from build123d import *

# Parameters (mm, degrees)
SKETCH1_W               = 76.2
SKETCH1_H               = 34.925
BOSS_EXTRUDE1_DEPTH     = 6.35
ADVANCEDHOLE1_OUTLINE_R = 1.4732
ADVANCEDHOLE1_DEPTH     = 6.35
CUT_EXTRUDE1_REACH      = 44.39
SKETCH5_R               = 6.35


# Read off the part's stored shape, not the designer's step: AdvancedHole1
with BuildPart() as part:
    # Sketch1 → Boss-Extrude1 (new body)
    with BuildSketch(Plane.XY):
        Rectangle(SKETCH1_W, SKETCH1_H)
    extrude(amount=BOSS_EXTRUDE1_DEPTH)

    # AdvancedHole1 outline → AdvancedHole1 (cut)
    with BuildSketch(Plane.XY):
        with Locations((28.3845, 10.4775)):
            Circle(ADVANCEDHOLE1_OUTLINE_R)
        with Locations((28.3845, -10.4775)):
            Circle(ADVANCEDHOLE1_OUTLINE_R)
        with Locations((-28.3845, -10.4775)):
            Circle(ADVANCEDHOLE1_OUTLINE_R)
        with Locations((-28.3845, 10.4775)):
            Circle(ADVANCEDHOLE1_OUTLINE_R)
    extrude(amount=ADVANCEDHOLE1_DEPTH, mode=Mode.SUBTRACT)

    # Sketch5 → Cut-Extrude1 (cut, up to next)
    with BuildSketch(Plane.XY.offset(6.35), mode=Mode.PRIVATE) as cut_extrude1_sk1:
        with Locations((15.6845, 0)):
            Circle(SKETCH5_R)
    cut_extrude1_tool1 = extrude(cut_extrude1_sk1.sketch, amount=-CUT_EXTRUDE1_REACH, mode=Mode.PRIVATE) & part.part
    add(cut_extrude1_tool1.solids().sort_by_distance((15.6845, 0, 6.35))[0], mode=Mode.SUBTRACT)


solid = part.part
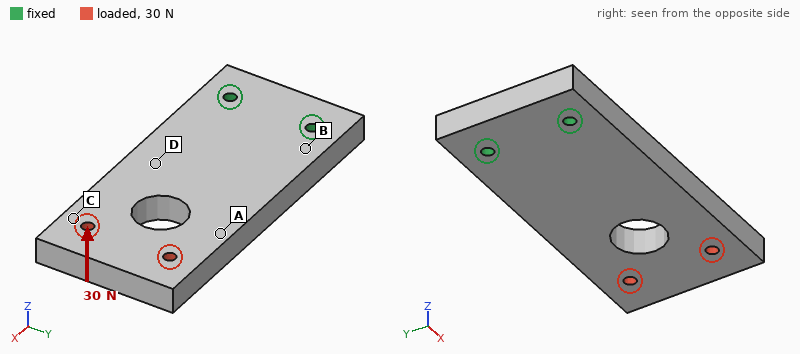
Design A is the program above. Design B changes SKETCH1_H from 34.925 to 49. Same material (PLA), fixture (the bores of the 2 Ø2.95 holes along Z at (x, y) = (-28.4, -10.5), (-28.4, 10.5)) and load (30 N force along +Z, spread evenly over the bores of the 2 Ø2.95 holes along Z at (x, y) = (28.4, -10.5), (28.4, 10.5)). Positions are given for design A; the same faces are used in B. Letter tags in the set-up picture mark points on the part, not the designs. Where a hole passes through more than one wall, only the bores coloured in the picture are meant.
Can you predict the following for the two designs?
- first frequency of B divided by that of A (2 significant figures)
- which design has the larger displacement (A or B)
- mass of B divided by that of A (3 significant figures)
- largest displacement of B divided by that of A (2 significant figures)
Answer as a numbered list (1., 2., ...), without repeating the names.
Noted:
1. 0.96
2. A
3. 1.43
4. 0.75
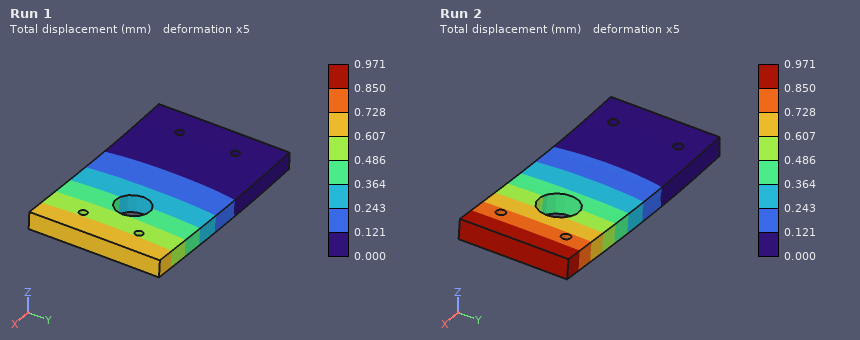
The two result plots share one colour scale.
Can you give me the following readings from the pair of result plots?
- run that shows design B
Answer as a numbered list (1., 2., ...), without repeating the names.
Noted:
1. Run 1
